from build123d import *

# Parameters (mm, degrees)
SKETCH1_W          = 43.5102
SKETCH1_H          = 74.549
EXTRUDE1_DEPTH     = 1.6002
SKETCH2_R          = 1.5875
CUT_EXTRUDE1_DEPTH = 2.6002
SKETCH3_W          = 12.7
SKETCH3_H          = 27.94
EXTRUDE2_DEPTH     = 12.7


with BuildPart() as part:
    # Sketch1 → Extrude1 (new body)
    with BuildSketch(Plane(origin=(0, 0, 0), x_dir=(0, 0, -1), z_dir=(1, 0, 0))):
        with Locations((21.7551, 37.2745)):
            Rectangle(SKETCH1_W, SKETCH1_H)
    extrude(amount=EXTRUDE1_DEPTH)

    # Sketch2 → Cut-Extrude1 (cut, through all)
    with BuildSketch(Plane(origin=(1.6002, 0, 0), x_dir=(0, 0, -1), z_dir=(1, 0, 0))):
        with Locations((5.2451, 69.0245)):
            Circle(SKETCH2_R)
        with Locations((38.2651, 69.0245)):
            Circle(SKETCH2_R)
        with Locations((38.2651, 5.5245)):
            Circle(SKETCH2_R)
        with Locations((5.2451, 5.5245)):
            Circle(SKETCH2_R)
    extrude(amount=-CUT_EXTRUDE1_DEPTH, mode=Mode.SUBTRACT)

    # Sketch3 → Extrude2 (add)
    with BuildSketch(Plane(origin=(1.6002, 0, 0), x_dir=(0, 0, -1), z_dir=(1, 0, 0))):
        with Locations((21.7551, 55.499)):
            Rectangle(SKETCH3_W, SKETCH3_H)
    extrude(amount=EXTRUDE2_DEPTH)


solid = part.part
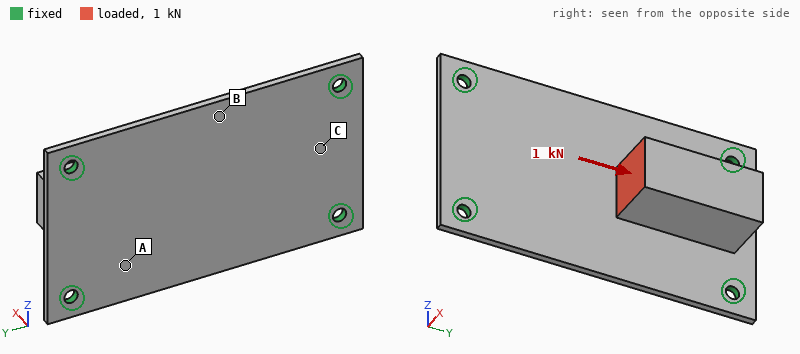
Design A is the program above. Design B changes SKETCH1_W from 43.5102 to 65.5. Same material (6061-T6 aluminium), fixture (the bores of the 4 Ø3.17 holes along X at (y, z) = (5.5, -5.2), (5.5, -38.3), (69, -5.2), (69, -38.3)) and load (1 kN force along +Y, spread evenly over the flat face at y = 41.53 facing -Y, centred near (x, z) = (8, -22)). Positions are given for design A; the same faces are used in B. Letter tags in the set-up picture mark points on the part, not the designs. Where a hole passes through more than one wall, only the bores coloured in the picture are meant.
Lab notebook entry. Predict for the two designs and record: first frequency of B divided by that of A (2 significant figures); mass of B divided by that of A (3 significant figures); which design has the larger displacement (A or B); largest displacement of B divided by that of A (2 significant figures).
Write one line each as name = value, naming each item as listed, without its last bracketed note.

first frequency of B divided by that of A = 1.0
mass of B divided by that of A = 1.27
which design has the larger displacement = A
largest displacement of B divided by that of A = 0.84
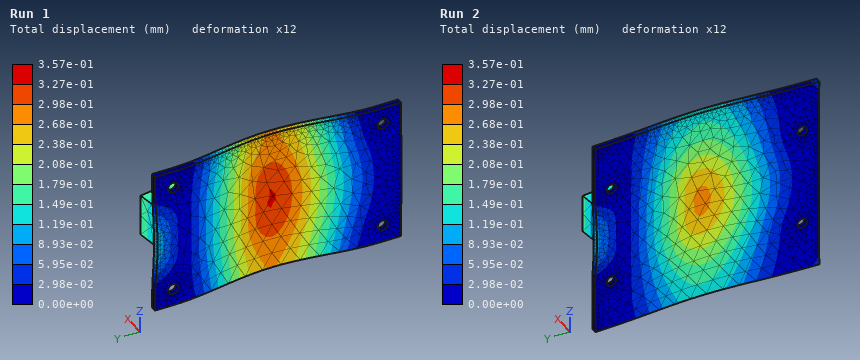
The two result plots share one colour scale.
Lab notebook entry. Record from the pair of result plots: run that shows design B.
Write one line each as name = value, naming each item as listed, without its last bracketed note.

run that shows design B = Run 2
